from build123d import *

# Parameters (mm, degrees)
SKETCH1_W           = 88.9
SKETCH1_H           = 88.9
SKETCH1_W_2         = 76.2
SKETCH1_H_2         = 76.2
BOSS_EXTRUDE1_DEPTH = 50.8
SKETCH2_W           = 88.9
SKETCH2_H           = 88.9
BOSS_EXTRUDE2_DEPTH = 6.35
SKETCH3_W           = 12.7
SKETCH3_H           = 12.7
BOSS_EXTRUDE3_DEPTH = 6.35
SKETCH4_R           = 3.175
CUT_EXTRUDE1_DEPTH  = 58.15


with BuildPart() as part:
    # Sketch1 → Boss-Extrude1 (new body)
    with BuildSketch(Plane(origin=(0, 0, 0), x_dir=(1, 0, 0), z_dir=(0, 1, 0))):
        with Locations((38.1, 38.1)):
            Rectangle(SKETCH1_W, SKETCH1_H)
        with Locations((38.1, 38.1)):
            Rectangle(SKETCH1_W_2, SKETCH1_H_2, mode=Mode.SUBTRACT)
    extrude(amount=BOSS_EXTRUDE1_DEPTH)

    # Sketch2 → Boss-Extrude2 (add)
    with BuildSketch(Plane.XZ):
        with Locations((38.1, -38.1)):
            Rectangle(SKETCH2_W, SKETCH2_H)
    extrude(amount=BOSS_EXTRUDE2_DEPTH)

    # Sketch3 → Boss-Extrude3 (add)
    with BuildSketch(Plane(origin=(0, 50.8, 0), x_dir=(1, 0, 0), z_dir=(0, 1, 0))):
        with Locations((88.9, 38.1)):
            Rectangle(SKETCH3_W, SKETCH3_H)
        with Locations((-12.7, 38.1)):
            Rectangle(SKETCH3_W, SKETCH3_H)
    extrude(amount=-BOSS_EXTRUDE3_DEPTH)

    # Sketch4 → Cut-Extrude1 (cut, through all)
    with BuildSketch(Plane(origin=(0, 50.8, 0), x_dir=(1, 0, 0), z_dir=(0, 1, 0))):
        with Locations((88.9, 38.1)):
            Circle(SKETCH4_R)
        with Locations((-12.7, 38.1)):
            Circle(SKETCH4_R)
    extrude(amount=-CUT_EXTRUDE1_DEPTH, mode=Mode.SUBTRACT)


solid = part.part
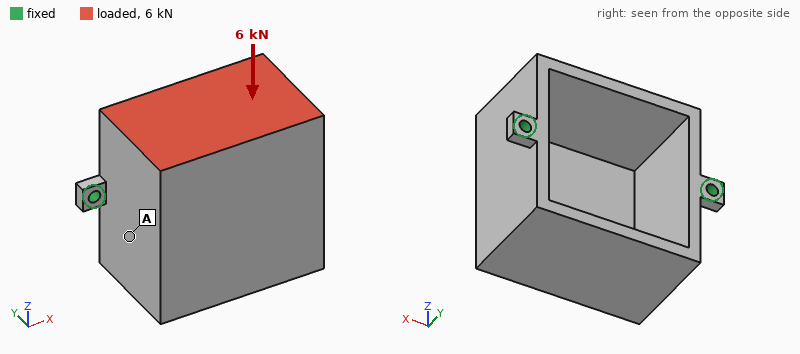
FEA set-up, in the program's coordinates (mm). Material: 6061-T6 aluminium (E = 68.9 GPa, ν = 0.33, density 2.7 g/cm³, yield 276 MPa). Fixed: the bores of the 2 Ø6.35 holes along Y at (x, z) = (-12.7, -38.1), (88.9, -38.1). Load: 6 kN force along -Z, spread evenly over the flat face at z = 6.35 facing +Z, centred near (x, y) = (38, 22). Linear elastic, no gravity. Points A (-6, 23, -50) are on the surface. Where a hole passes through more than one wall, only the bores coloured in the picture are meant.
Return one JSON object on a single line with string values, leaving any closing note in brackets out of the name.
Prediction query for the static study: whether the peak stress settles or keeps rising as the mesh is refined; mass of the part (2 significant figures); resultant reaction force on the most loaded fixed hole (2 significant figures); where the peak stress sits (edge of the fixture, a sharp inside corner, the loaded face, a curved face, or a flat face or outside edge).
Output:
{"whether the peak stress settles or keeps rising as the mesh is refined": "keeps rising", "mass of the part": "430 g", "resultant reaction force on the most loaded fixed hole": "3.0 kN", "where the peak stress sits": "edge of the fixture"}
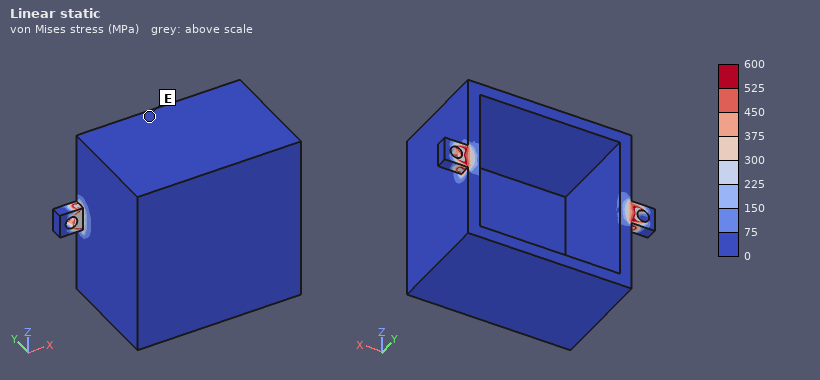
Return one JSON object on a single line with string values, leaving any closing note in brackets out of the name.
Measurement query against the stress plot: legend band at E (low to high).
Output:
{"legend band at E": "0 to 75 MPa"}
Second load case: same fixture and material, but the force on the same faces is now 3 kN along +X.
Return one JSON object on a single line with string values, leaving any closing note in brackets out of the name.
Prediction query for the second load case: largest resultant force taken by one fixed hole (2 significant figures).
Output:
{"largest resultant force taken by one fixed hole": "2.0 kN"}
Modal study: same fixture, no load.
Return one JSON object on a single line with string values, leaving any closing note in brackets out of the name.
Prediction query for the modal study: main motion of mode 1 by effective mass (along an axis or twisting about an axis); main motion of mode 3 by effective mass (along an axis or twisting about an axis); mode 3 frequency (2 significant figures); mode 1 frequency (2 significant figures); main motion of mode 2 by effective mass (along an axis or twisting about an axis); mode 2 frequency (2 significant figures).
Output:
{"main motion of mode 1 by effective mass": "along Z", "main motion of mode 3 by effective mass": "twisting about Y", "mode 3 frequency": "1400 Hz", "mode 1 frequency": "440 Hz", "main motion of mode 2 by effective mass": "along X", "mode 2 frequency": "1300 Hz"}
